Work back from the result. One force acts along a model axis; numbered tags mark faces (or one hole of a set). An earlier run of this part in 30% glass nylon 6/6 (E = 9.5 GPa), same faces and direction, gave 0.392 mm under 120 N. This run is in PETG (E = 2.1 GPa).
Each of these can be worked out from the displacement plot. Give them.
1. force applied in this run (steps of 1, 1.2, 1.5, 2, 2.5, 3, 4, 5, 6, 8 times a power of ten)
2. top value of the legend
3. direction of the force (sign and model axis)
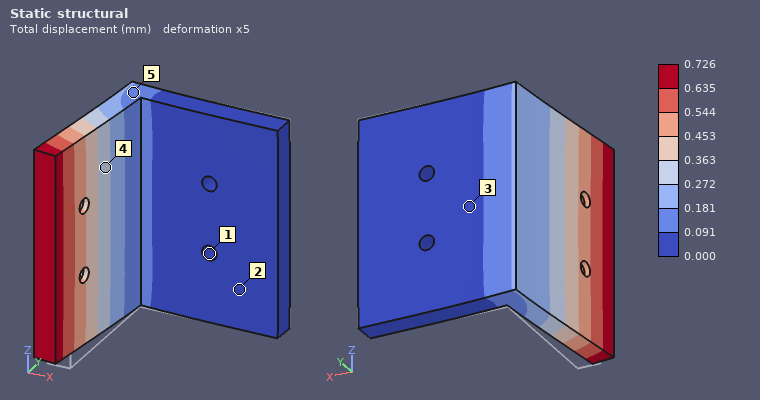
50 N
0.726 mm
-X
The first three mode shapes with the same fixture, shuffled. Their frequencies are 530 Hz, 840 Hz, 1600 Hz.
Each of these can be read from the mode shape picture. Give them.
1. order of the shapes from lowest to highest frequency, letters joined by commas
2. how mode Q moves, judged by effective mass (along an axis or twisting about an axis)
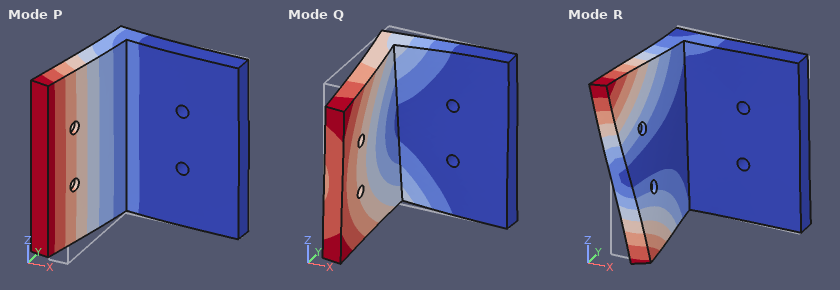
P, Q, R
along Z
